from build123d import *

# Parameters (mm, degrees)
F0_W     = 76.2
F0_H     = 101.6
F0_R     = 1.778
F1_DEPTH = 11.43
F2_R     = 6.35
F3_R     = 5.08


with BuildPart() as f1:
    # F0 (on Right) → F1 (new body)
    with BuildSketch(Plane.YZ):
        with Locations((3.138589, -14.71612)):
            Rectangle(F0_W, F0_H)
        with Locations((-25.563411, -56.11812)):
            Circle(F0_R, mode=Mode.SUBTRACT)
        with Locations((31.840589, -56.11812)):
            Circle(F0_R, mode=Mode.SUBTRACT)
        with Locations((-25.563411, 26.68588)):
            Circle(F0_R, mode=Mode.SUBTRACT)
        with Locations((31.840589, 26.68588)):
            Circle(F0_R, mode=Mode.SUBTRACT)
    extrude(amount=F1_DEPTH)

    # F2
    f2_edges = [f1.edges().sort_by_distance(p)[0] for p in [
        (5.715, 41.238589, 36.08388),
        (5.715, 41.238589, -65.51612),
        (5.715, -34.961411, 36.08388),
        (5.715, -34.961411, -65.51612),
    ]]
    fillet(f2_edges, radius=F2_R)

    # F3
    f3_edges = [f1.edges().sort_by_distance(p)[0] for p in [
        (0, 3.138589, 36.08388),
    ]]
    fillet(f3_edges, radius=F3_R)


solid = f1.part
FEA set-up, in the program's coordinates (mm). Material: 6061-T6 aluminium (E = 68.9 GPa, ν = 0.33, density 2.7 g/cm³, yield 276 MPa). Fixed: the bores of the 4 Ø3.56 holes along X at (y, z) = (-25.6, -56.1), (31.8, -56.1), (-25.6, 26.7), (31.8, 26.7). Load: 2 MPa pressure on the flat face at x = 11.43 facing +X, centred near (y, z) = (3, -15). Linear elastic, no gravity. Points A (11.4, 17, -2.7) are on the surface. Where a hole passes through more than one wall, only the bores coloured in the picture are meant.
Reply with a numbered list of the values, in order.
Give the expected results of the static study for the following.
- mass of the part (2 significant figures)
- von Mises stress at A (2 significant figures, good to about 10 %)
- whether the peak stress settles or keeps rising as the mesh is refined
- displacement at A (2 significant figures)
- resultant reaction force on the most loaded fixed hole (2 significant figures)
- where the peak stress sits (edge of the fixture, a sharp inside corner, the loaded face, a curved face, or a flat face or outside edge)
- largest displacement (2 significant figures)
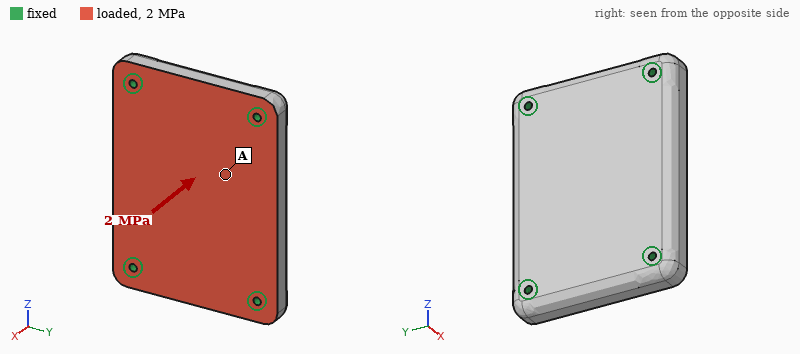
1. 230 g
2. 25 MPa
3. keeps rising
4. 56 µm
5. 3.8 kN
6. edge of the fixture
7. 63 µm
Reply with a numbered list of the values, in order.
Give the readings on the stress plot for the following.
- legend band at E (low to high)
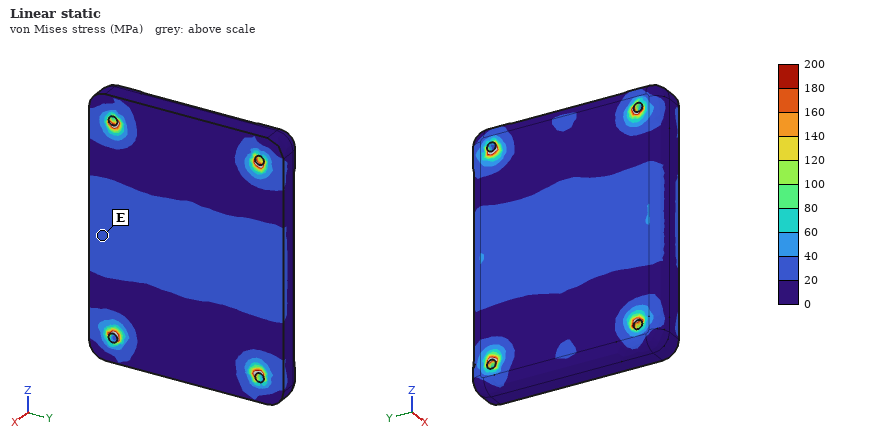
1. 20 to 40 MPa
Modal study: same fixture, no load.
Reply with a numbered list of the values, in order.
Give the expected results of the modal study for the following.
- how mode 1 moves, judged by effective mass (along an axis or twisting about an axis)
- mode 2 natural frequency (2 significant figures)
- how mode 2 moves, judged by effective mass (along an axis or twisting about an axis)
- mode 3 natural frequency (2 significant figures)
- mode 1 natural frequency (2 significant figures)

1. along X
2. 8600 Hz
3. twisting about Z
4. 12 kHz
5. 5800 Hz
